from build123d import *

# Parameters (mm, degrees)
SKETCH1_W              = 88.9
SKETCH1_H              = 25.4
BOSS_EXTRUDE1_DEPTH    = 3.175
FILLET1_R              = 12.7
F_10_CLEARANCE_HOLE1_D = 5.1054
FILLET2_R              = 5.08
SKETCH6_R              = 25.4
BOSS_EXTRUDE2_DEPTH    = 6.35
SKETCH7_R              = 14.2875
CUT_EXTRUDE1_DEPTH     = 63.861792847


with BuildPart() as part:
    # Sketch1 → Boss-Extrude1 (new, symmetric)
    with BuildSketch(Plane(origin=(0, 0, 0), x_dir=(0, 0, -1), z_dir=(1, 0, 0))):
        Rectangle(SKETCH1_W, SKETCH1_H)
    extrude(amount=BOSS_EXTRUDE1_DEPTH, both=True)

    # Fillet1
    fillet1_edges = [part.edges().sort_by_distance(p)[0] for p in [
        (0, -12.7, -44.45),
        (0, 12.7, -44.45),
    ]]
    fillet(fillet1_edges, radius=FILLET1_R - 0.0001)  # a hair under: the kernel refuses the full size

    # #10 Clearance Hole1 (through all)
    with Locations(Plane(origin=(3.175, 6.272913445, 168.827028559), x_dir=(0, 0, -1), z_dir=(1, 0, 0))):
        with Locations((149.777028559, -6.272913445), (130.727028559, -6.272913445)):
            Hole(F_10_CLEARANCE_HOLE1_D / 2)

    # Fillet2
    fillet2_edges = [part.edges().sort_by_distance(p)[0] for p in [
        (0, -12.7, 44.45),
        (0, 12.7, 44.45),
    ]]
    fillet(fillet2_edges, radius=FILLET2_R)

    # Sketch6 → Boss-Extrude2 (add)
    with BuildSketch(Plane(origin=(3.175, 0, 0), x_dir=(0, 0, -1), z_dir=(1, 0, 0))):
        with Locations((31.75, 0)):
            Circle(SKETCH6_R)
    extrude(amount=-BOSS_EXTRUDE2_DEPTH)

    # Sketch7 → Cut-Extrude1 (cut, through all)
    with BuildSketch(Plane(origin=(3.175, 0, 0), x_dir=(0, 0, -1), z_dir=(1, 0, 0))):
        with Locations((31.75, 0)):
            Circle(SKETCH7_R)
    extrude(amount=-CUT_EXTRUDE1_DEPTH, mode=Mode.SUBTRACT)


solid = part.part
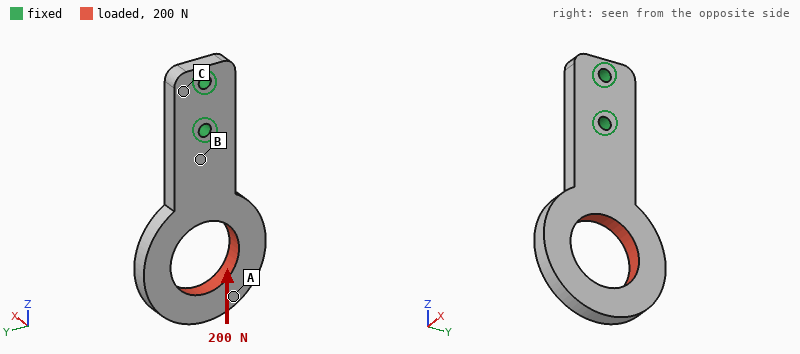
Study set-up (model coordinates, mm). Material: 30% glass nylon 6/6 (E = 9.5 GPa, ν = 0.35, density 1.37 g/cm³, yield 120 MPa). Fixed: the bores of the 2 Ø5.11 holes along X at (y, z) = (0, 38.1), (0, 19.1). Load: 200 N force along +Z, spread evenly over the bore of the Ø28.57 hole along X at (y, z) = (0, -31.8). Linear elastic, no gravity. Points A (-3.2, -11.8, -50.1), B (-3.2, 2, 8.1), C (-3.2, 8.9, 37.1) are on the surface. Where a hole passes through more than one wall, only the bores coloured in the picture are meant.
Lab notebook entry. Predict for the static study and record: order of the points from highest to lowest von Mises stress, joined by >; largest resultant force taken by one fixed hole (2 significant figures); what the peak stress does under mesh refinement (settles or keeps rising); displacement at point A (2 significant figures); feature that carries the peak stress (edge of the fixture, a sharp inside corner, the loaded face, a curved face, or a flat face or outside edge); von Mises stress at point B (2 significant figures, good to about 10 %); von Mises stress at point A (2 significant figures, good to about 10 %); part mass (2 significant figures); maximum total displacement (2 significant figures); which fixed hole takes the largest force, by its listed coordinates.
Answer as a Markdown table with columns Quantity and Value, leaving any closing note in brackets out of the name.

| Quantity | Value |
|---|---|
| order of the points from highest to lowest von Mises stress, joined by > | B > A > C |
| largest resultant force taken by one fixed hole | 160 N |
| what the peak stress does under mesh refinement | keeps rising |
| displacement at point A | 15 µm |
| feature that carries the peak stress | a sharp inside corner |
| von Mises stress at point B | 1.5 MPa |
| von Mises stress at point A | 0.75 MPa |
| part mass | 23 g |
| maximum total displacement | 18 µm |
| which fixed hole takes the largest force, by its listed coordinates | (0, 19.1) |
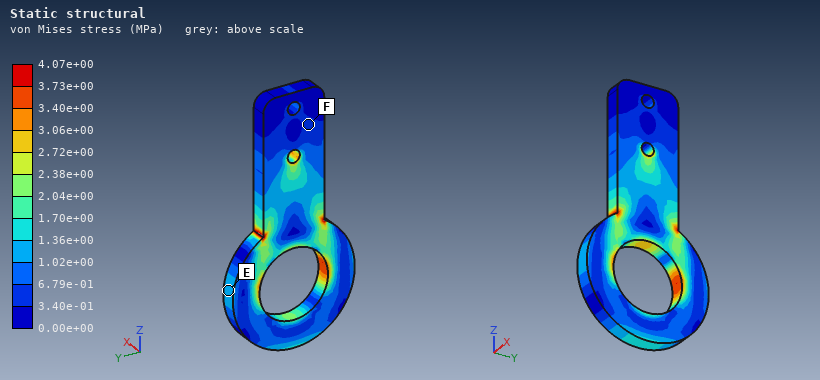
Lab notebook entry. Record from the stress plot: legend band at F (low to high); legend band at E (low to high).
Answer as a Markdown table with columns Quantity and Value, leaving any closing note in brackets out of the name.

| Quantity | Value |
|---|---|
| legend band at F | 3.40e-01 to 6.79e-01 MPa |
| legend band at E | 1.02e+00 to 1.36e+00 MPa |
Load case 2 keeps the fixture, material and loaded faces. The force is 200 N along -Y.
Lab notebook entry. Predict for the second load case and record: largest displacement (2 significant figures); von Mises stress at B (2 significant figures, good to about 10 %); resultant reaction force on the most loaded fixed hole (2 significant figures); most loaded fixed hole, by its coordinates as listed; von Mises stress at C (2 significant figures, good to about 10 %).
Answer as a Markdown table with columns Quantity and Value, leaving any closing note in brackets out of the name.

| Quantity | Value |
|---|---|
| largest displacement | 0.37 mm |
| von Mises stress at B | 3.6 MPa |
| resultant reaction force on the most loaded fixed hole | 560 N |
| most loaded fixed hole, by its coordinates as listed | (0, 19.1) |
| von Mises stress at C | 2.3 MPa |
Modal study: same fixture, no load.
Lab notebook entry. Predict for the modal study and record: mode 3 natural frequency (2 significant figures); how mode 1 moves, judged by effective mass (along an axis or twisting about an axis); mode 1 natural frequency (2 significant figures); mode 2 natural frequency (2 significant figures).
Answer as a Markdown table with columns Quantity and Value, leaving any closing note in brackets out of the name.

| Quantity | Value |
|---|---|
| mode 3 natural frequency | 1200 Hz |
| how mode 1 moves, judged by effective mass | along X |
| mode 1 natural frequency | 440 Hz |
| mode 2 natural frequency | 1200 Hz |
